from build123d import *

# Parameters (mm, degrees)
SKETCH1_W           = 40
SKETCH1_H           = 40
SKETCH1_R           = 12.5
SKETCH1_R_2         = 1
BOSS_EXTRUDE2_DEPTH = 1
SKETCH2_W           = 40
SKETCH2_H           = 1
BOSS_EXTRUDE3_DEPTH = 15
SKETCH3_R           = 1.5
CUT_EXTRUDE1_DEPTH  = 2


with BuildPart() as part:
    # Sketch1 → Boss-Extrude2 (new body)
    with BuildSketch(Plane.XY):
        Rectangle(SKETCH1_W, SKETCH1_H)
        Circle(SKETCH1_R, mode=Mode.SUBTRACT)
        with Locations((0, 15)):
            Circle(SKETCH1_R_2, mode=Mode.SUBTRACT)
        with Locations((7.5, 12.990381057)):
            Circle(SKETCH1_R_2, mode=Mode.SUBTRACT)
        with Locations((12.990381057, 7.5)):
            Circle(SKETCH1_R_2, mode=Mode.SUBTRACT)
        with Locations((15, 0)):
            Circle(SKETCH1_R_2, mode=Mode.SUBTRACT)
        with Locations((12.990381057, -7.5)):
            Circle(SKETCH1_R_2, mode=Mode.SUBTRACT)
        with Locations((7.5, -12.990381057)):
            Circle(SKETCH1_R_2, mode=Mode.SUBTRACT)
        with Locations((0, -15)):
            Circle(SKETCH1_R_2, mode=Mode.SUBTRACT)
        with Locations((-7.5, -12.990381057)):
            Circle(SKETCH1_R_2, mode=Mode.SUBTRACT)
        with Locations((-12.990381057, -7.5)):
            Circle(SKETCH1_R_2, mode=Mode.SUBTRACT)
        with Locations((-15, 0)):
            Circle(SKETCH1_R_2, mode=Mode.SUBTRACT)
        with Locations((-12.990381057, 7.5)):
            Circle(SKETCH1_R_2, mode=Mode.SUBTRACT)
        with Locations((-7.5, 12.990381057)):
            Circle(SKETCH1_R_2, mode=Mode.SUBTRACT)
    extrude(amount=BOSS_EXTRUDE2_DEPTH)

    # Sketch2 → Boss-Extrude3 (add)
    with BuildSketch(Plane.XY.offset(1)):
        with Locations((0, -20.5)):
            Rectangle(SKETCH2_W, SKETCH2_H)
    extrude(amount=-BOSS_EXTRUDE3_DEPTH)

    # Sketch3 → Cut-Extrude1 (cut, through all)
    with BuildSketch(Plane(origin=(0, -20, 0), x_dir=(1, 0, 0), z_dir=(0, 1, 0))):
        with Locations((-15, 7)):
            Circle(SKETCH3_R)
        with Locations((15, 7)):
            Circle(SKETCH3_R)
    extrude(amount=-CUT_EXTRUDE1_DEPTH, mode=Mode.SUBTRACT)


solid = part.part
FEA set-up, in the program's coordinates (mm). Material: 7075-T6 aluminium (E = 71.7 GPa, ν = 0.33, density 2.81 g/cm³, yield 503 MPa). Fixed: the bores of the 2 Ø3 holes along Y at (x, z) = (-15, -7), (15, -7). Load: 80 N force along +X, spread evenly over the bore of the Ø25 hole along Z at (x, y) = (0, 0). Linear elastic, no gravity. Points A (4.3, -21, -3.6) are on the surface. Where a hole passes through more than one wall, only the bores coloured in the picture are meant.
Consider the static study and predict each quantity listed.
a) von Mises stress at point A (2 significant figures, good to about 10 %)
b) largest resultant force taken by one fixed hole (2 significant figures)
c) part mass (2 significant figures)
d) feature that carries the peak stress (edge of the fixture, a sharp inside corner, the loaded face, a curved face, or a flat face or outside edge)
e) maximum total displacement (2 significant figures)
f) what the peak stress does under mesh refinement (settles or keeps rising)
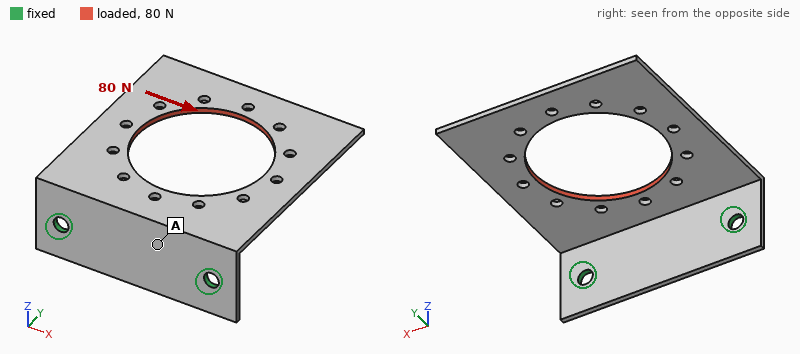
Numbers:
17 MPa
69 N
4.7 g
edge of the fixture
0.23 mm
keeps rising
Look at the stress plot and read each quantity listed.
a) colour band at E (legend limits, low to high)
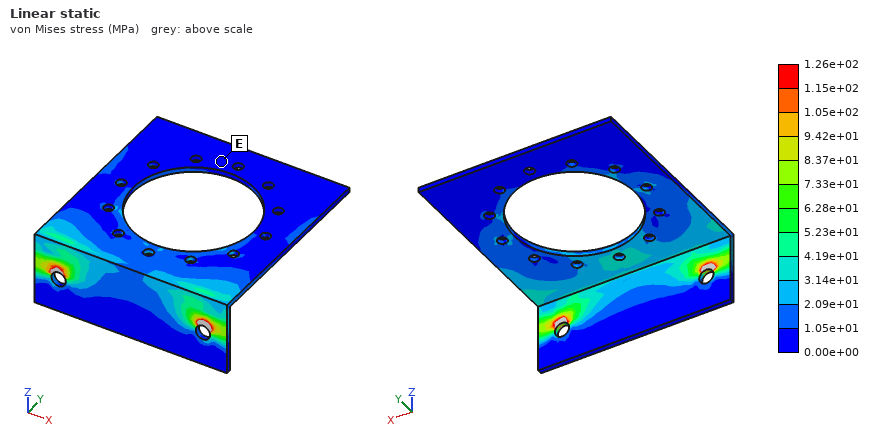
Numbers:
0.00e+00 to 1.05e+01 MPa
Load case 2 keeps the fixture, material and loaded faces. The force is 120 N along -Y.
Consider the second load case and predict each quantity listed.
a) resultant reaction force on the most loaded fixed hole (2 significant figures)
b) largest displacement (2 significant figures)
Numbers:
60 N
0.60 mm
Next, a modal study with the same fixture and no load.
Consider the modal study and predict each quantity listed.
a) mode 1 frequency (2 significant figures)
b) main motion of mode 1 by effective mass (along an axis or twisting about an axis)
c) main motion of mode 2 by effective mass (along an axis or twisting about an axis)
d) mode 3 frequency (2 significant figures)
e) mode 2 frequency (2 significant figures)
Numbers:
370 Hz
along Z
twisting about Y
2200 Hz
920 Hz
